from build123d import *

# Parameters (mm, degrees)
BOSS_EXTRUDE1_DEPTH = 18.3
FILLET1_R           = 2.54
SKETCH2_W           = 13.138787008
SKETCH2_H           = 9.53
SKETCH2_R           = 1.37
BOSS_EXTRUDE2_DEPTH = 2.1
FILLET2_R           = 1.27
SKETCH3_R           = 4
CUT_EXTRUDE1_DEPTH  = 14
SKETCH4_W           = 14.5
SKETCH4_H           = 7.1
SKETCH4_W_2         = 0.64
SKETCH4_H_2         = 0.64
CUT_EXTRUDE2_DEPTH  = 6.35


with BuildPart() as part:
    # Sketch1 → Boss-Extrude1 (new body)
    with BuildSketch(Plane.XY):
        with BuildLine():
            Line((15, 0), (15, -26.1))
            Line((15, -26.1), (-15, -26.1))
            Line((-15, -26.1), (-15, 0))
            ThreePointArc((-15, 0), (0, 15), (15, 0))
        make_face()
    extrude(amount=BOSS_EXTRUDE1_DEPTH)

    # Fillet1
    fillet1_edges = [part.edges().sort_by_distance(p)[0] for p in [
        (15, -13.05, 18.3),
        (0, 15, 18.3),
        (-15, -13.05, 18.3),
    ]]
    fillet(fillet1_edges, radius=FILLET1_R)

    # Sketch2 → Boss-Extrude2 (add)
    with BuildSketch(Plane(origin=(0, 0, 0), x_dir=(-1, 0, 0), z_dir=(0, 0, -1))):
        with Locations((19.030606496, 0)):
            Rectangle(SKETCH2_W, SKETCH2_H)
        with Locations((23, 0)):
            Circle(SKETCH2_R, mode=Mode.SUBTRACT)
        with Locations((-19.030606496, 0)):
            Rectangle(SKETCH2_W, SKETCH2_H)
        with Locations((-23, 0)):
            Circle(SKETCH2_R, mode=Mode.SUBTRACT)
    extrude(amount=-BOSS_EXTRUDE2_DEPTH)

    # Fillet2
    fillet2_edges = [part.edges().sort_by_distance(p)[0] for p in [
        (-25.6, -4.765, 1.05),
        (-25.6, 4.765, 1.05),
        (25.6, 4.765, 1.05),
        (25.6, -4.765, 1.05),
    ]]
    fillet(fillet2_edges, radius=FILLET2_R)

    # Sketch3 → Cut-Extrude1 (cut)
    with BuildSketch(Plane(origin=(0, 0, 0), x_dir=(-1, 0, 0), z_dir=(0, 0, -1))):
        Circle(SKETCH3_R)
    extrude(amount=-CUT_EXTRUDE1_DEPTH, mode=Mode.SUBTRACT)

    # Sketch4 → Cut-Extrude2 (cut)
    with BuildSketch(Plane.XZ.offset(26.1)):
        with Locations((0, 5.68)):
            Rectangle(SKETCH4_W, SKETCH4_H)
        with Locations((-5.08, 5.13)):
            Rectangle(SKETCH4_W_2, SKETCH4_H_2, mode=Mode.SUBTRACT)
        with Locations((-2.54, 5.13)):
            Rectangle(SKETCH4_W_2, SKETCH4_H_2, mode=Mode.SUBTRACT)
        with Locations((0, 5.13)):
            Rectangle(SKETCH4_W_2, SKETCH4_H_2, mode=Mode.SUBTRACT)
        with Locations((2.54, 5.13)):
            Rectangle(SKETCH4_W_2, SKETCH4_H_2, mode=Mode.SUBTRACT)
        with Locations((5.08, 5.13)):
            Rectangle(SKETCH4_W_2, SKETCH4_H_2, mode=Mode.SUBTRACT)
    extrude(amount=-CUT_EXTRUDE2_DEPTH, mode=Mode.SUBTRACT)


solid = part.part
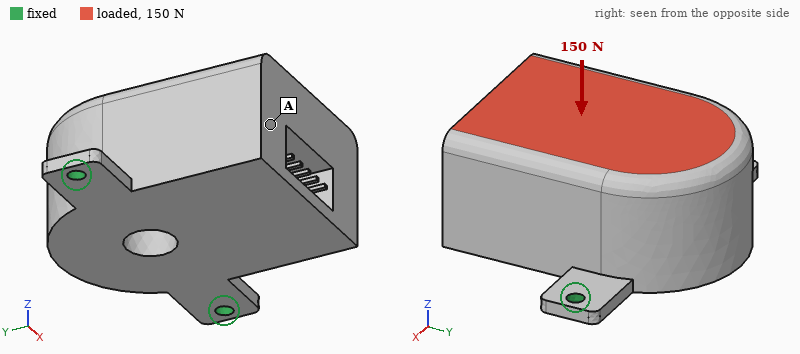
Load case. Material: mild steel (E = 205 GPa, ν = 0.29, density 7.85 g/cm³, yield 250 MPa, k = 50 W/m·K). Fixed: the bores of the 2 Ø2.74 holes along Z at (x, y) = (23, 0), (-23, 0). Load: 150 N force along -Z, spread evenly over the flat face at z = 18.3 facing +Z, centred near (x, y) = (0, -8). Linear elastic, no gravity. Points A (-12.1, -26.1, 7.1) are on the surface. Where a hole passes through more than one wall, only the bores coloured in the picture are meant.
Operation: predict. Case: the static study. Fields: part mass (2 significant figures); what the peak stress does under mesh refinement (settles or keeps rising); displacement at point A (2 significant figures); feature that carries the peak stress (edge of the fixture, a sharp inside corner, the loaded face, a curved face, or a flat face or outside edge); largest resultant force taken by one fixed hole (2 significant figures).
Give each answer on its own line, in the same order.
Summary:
150 g
keeps rising
53 µm
edge of the fixture
84 N
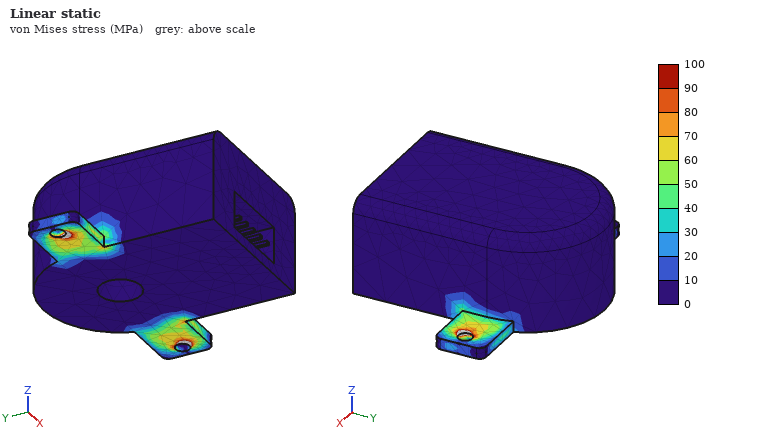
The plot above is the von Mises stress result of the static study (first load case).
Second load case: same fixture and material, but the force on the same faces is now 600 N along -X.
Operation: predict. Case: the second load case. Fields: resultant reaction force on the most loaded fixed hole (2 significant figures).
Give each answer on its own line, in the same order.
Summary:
420 N
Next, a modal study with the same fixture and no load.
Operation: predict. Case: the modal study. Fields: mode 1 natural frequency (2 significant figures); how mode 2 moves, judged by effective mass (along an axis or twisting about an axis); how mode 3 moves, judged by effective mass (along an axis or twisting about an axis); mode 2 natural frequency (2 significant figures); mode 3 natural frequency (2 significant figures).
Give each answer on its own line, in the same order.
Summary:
630 Hz
along Z
along X
3100 Hz
3900 Hz
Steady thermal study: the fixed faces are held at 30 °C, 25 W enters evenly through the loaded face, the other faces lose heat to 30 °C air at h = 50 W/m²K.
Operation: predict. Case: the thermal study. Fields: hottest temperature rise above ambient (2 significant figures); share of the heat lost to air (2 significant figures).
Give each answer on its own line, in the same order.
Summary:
68 K
54 %
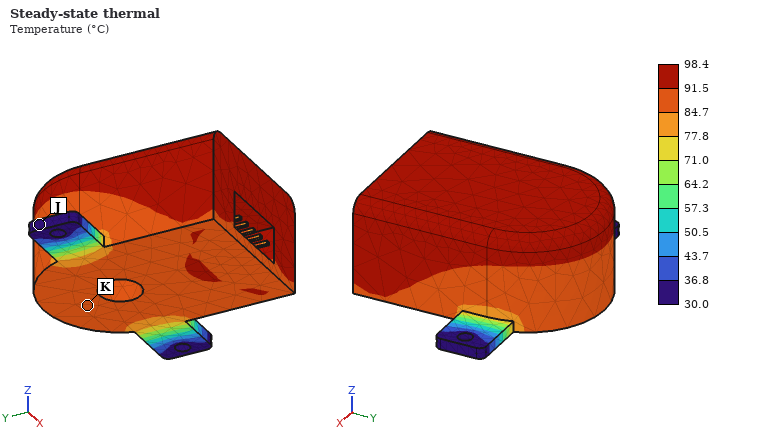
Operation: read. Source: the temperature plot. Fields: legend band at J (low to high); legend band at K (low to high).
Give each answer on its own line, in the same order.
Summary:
30.0 to 36.8 °C
84.7 to 91.5 °C
